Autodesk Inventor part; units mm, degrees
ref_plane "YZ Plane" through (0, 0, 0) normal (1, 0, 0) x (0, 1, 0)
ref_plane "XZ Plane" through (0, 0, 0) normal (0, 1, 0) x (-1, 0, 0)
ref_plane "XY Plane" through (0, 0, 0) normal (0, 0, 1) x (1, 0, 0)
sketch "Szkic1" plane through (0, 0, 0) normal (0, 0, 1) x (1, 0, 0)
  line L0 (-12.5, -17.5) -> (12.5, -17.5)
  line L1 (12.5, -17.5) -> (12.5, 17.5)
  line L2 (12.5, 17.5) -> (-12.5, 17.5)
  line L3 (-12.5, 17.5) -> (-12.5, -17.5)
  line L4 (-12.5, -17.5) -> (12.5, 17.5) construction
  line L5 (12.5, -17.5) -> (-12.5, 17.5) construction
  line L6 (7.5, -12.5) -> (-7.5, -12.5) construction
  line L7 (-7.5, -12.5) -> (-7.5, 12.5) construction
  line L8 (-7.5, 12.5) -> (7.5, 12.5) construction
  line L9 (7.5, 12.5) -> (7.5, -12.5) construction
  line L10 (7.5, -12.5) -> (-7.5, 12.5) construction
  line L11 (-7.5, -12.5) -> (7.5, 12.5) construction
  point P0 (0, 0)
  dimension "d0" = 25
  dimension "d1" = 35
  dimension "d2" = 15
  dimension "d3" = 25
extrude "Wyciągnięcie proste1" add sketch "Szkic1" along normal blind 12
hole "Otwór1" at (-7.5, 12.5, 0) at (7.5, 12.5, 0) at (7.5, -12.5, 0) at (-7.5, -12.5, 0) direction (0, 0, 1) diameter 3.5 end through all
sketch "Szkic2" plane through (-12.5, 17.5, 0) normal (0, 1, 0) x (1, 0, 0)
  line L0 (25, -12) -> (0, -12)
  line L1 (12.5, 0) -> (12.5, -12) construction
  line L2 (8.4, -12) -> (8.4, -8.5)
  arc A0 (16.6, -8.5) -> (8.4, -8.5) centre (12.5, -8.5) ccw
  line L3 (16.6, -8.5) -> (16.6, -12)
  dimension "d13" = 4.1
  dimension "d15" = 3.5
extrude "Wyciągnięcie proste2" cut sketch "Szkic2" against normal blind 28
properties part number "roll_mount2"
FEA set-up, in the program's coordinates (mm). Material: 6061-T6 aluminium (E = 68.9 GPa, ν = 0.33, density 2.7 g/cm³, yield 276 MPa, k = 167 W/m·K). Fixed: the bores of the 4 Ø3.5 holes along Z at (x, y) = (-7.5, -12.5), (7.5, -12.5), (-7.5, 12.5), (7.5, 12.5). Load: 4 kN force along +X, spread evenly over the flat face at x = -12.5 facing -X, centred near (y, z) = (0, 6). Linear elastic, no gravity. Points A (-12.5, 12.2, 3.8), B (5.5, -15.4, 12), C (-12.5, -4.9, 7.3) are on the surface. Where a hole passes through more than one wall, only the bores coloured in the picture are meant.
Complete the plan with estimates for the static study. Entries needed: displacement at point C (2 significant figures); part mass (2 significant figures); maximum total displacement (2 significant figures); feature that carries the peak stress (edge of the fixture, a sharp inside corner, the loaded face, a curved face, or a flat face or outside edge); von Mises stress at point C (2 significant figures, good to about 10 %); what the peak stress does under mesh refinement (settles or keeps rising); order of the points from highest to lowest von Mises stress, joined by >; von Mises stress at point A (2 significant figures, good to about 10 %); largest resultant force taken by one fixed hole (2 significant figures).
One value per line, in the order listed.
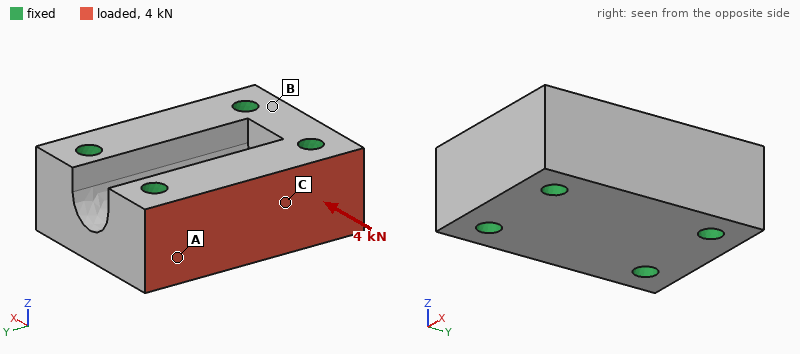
3.5 µm
23 g
5.4 µm
edge of the fixture
12 MPa
keeps rising
A > C > B
19 MPa
1.7 kN
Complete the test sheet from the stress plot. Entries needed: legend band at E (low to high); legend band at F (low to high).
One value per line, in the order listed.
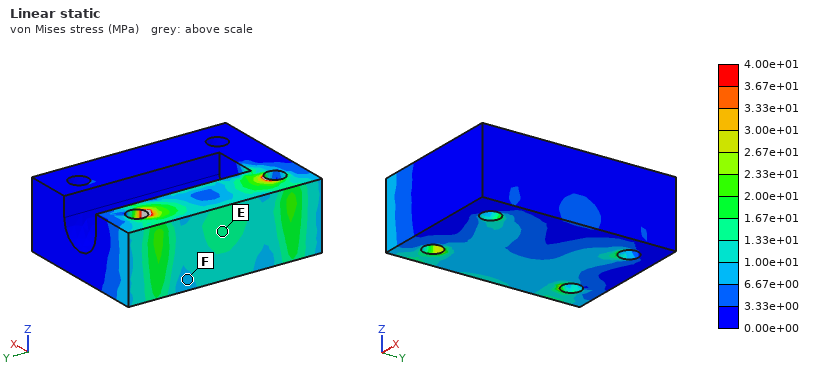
1.33e+01 to 1.67e+01 MPa
6.67e+00 to 1.00e+01 MPa
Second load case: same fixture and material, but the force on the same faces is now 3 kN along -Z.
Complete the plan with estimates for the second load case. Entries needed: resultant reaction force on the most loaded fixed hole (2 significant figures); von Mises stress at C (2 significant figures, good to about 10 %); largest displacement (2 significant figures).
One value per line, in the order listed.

1.6 kN
25 MPa
8.5 µm
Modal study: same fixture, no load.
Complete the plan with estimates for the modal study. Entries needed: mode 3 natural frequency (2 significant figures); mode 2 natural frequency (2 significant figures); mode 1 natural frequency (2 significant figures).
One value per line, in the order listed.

55 kHz
51 kHz
50 kHz
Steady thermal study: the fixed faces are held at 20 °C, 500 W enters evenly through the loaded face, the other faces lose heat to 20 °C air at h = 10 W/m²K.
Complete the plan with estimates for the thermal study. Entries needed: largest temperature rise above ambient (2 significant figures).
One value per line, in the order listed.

75 K
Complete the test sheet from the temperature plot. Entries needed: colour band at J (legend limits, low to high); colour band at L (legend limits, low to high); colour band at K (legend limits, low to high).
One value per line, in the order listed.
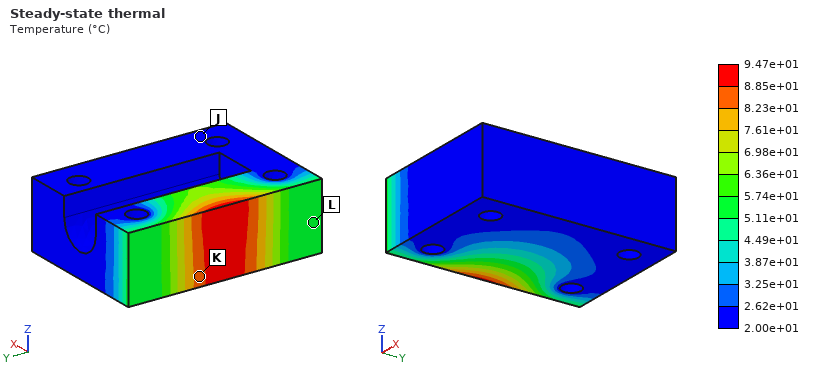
2.00e+01 to 2.62e+01 °C
5.11e+01 to 5.74e+01 °C
8.23e+01 to 8.85e+01 °C
